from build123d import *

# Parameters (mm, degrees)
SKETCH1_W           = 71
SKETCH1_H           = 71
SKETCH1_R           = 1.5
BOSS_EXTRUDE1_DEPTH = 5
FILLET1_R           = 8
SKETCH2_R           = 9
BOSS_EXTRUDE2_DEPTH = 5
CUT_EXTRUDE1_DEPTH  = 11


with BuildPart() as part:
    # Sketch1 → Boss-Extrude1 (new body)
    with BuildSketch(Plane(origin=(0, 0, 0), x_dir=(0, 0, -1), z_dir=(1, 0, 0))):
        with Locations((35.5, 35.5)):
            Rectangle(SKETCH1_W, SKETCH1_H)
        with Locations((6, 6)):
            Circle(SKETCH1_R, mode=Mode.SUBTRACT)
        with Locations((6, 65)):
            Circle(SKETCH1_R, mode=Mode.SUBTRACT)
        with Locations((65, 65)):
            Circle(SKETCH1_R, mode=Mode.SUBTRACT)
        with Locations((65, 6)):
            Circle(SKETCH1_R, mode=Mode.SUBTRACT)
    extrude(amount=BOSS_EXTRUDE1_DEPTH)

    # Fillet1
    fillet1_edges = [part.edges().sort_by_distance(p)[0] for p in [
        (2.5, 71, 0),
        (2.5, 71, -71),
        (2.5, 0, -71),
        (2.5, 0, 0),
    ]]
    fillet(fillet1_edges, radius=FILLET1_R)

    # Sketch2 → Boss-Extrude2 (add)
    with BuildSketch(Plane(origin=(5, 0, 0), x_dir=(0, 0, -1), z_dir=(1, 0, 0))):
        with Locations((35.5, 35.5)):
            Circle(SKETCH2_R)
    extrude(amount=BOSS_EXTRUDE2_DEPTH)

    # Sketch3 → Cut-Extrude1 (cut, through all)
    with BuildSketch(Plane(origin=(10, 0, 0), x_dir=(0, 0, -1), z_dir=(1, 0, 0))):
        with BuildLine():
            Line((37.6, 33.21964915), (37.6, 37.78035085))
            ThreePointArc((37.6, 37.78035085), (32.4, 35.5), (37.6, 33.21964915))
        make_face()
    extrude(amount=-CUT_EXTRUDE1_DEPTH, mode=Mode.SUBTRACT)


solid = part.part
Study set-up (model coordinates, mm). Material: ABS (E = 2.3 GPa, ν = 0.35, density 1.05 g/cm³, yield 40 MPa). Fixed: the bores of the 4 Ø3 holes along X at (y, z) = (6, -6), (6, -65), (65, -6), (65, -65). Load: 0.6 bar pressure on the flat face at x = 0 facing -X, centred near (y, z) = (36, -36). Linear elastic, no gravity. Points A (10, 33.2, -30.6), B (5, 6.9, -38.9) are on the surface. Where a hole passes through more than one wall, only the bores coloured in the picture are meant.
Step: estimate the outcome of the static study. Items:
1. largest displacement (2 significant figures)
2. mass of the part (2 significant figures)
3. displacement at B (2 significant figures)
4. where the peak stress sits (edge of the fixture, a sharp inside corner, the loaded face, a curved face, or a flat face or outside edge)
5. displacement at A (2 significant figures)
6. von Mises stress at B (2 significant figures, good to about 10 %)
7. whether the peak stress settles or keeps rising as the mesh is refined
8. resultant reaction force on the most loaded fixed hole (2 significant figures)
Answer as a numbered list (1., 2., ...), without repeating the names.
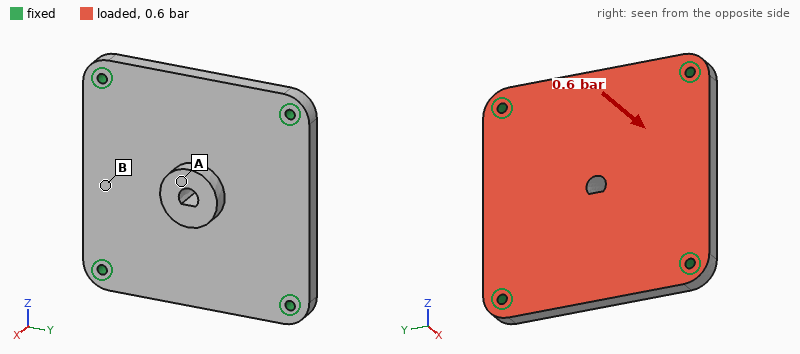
1. 0.21 mm
2. 27 g
3. 0.13 mm
4. edge of the fixture
5. 0.21 mm
6. 2.7 MPa
7. keeps rising
8. 74 N
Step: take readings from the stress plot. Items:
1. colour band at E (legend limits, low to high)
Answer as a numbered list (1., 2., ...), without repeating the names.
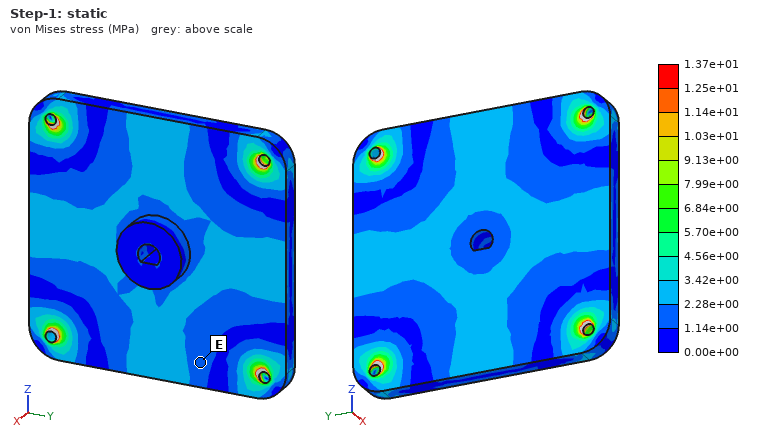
1. 1.14e+00 to 2.28e+00 MPa
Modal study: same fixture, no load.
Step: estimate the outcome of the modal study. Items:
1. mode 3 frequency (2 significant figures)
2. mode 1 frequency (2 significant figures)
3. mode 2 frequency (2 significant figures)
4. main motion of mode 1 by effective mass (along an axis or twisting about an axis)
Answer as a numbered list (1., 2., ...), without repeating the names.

1. 2200 Hz
2. 1300 Hz
3. 2200 Hz
4. along X
